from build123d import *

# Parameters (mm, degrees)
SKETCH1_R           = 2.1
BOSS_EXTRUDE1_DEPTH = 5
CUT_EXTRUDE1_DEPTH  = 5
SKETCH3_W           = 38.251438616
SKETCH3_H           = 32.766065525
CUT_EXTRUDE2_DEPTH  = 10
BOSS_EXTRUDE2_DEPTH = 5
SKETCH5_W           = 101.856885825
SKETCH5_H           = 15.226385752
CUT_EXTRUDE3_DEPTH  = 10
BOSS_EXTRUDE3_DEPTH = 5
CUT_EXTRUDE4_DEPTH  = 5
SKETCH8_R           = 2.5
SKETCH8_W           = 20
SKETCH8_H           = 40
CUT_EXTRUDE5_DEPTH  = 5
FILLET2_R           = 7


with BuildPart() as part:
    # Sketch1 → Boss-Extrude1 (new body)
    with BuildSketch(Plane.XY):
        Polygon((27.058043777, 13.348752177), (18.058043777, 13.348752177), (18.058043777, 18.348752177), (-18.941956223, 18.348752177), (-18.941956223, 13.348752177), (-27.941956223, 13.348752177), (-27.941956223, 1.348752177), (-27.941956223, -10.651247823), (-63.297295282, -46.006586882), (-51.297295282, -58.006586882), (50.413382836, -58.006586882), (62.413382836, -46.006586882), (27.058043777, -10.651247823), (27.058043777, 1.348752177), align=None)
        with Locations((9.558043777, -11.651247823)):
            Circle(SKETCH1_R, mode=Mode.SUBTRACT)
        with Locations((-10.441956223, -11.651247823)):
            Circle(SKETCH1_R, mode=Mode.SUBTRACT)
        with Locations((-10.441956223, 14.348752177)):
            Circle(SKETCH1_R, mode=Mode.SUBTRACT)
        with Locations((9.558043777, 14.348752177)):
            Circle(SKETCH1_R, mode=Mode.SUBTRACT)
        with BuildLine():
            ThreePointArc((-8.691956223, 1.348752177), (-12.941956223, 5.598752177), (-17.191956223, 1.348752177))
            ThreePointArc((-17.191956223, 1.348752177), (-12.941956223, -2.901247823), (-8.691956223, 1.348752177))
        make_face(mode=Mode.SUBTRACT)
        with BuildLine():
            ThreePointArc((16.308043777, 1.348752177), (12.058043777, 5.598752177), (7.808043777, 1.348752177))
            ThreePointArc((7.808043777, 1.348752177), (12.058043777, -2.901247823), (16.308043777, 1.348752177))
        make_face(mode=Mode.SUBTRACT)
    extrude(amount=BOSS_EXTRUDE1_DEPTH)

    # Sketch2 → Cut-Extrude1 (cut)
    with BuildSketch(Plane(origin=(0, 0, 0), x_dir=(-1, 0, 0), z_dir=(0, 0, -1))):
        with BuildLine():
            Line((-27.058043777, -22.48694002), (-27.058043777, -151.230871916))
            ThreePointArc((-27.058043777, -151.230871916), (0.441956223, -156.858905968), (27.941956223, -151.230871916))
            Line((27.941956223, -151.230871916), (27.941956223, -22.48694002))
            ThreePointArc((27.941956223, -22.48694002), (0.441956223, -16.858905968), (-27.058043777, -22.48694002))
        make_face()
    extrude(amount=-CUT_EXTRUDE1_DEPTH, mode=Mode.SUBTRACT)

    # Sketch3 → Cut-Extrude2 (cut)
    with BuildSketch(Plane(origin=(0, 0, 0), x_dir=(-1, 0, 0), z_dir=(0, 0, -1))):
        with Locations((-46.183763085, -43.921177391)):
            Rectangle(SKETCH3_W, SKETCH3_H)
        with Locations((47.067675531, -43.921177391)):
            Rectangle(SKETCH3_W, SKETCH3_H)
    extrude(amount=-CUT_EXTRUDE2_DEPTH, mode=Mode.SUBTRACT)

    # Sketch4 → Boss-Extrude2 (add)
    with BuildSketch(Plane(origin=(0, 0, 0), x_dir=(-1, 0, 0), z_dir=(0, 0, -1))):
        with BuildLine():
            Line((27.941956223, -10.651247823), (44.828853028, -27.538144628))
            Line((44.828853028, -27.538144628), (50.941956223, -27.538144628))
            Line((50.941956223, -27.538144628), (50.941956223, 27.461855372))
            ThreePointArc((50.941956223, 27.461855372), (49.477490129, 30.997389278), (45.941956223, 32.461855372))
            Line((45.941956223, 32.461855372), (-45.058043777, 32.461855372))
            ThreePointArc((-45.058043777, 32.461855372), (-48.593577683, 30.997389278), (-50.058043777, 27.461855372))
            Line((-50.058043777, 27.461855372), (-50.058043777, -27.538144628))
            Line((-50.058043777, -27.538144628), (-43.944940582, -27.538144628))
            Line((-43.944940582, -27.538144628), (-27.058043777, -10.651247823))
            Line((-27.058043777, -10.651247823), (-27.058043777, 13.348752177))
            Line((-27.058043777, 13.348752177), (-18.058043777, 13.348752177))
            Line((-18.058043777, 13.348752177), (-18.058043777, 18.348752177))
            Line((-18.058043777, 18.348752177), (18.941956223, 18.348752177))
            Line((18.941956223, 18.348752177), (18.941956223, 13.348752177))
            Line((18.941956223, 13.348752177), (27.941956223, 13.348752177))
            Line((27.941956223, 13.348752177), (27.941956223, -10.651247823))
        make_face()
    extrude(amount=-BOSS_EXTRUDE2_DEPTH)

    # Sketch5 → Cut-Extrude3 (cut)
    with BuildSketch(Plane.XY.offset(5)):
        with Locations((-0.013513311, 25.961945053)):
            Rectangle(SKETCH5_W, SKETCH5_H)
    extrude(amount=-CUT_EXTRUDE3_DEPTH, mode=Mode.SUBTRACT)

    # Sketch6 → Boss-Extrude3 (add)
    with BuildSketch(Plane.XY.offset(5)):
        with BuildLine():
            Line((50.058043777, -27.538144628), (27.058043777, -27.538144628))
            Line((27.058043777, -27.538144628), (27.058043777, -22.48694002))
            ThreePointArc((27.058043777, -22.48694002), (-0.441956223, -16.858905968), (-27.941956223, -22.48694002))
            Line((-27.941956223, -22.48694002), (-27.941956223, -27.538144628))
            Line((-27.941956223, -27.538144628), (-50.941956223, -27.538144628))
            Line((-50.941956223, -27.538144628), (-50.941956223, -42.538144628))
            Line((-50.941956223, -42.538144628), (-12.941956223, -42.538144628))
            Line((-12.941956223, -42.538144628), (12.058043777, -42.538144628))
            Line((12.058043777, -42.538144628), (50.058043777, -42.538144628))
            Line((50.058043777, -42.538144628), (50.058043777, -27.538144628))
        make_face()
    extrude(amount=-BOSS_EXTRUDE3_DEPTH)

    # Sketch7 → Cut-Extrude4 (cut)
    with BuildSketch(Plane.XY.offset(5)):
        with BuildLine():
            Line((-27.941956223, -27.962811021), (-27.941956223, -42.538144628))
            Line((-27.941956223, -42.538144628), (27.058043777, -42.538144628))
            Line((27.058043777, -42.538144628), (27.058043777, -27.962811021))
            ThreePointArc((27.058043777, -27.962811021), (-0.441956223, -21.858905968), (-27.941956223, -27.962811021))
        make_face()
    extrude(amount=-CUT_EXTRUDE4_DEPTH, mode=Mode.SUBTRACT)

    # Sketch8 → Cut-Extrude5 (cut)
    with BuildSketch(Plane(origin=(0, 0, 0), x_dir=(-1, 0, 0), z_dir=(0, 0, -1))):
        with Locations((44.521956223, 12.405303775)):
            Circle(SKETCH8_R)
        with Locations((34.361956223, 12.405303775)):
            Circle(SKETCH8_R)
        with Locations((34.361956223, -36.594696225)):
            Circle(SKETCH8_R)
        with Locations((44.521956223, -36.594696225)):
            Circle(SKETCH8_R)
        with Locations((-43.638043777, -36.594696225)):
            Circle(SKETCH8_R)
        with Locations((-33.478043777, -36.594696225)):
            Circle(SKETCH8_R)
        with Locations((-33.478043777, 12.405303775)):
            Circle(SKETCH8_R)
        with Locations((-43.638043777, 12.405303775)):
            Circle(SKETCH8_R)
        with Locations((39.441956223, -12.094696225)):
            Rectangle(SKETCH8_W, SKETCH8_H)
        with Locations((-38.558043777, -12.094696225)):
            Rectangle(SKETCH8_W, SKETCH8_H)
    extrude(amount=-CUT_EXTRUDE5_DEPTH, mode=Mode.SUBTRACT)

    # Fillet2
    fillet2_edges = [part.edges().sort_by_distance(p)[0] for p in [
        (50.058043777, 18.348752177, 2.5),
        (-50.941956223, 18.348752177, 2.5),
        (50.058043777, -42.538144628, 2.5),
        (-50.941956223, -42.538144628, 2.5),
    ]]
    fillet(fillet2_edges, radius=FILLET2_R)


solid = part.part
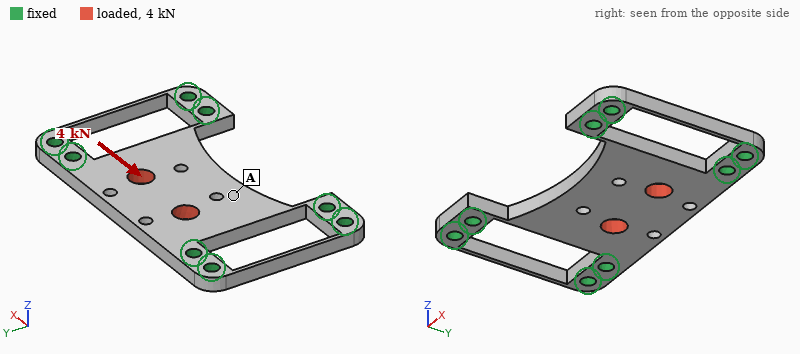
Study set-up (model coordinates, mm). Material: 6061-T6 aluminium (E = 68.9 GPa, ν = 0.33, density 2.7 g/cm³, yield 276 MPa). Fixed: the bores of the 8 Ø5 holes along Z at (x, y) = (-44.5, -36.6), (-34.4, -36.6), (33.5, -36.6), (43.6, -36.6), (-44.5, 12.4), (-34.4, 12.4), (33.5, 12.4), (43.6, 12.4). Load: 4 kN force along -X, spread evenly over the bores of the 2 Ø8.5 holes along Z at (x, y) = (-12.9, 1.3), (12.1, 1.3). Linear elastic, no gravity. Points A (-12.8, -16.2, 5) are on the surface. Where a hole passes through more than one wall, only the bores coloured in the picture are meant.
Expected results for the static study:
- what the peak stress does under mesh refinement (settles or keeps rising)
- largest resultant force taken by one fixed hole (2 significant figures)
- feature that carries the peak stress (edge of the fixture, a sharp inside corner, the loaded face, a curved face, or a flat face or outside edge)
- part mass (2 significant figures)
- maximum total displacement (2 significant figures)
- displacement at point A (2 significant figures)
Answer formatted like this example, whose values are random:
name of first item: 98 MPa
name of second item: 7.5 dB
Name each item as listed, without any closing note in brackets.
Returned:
what the peak stress does under mesh refinement: keeps rising
largest resultant force taken by one fixed hole: 1.9 kN
feature that carries the peak stress: a sharp inside corner
part mass: 43 g
maximum total displacement: 16 µm
displacement at point A: 15 µm
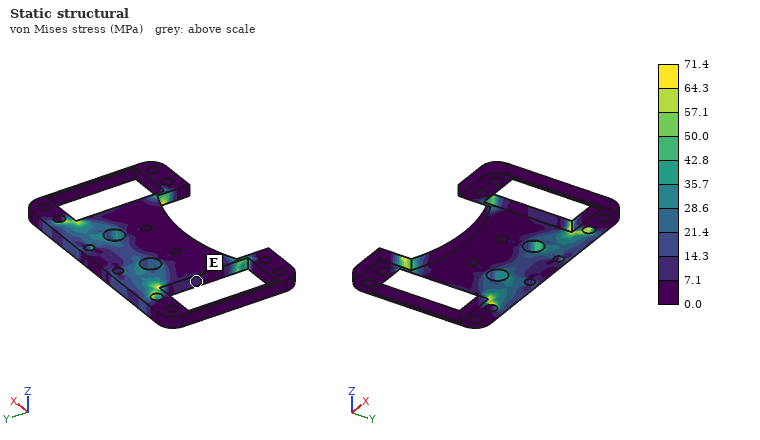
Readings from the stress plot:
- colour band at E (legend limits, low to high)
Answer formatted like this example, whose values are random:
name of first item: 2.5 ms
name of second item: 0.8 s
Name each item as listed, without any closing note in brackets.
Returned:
colour band at E: 7.1 to 14.3 MPa
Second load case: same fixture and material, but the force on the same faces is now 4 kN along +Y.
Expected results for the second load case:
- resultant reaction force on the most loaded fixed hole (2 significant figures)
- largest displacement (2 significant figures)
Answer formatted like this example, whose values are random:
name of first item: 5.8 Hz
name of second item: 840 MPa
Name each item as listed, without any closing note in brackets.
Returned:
resultant reaction force on the most loaded fixed hole: 1.7 kN
largest displacement: 26 µm
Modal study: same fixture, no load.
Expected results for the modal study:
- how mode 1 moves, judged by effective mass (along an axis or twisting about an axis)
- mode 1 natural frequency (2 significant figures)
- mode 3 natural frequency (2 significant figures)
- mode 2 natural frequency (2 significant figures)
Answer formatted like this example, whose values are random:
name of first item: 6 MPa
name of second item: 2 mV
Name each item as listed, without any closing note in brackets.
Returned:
how mode 1 moves, judged by effective mass: along Z
mode 1 natural frequency: 3700 Hz
mode 3 natural frequency: 4500 Hz
mode 2 natural frequency: 4500 Hz
